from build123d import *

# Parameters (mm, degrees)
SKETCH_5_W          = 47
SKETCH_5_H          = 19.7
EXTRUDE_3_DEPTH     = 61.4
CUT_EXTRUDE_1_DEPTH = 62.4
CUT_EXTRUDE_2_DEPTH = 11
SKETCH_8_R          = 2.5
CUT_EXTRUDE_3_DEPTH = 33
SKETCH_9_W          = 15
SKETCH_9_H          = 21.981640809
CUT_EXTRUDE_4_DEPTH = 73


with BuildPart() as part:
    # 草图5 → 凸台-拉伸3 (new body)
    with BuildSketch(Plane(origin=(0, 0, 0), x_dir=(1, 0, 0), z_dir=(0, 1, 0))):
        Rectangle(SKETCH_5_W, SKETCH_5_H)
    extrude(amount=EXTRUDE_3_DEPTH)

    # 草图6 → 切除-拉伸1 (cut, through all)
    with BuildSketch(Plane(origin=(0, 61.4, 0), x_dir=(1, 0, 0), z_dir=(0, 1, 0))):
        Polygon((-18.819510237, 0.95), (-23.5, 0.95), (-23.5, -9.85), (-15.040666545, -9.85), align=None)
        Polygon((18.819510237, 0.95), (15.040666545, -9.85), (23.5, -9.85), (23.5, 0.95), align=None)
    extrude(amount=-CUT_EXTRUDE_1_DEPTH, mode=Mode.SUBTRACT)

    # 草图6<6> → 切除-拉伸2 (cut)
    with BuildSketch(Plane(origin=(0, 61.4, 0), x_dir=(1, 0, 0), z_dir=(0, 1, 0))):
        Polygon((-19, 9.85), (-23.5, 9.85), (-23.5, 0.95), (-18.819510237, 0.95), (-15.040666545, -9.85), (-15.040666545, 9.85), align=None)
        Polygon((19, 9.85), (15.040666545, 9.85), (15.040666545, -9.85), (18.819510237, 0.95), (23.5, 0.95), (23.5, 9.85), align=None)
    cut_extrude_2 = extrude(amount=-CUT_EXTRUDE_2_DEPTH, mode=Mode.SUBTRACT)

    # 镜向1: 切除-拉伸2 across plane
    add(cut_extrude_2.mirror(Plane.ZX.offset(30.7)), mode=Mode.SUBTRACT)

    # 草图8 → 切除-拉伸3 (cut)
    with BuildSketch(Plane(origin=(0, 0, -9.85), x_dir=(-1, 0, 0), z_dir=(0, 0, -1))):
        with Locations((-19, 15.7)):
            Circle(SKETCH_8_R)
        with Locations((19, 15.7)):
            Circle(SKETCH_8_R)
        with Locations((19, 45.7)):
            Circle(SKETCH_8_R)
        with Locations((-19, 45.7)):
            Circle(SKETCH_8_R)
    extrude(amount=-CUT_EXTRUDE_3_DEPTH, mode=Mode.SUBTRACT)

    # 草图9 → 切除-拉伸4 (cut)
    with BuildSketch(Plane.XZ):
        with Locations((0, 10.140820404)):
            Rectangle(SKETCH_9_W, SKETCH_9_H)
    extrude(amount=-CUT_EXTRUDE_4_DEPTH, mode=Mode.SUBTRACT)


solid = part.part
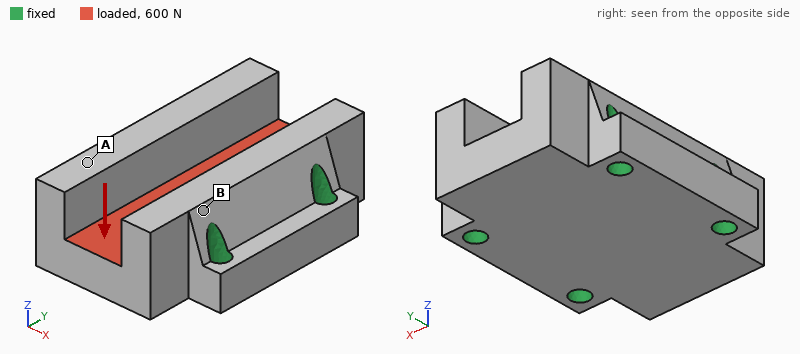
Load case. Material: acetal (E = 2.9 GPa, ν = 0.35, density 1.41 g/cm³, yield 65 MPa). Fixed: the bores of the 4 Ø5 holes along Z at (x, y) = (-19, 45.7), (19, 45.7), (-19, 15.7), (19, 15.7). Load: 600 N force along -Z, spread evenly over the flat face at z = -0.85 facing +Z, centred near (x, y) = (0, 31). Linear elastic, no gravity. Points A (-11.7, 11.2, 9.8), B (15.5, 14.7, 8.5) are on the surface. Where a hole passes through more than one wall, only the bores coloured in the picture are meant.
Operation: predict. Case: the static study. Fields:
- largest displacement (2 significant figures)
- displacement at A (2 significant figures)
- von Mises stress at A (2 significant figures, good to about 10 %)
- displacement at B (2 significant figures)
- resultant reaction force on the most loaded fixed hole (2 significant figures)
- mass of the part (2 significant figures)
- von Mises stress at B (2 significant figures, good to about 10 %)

25 µm
13 µm
0.49 MPa
9.3 µm
160 N
47 g
1.1 MPa
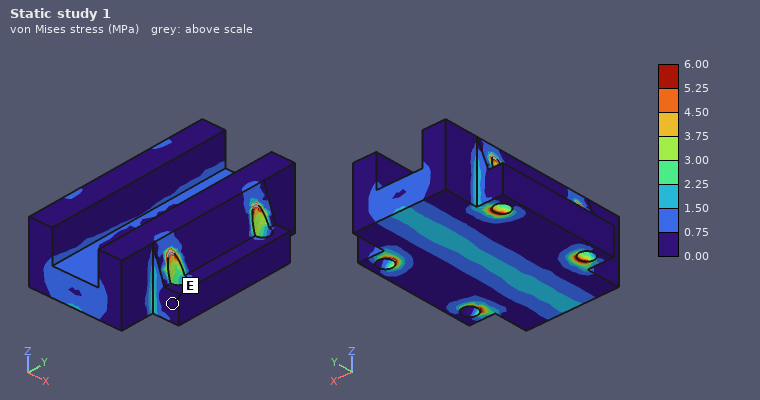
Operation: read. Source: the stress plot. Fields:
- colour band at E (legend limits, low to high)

0.00 to 0.75 MPa
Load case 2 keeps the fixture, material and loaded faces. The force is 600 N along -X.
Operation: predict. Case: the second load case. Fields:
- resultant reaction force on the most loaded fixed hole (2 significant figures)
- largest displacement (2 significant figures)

150 N
8.3 µm
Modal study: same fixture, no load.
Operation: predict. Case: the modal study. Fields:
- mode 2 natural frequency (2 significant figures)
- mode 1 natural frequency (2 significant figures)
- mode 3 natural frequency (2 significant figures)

5800 Hz
5800 Hz
7700 Hz
